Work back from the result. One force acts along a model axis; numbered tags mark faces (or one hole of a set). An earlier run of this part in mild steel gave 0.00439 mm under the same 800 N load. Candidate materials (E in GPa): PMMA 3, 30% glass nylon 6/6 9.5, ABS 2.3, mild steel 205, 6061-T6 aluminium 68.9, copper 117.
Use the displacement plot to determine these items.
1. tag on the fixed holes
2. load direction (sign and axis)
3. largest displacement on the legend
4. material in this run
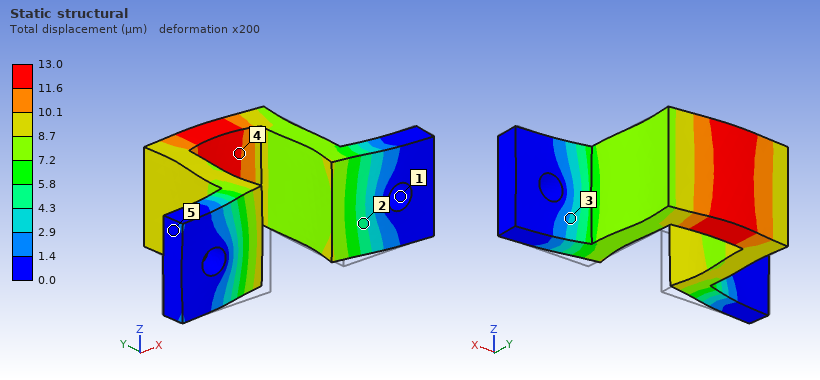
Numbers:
1
+Y
13.0 µm
6061-T6 aluminium
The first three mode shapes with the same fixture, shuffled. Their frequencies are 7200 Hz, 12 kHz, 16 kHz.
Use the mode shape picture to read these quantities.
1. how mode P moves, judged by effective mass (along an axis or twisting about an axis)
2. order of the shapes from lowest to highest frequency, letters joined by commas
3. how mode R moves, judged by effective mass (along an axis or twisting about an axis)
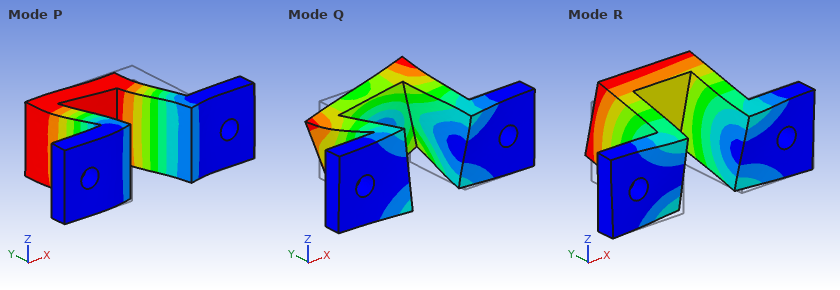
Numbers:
along X
R, P, Q
along Z
